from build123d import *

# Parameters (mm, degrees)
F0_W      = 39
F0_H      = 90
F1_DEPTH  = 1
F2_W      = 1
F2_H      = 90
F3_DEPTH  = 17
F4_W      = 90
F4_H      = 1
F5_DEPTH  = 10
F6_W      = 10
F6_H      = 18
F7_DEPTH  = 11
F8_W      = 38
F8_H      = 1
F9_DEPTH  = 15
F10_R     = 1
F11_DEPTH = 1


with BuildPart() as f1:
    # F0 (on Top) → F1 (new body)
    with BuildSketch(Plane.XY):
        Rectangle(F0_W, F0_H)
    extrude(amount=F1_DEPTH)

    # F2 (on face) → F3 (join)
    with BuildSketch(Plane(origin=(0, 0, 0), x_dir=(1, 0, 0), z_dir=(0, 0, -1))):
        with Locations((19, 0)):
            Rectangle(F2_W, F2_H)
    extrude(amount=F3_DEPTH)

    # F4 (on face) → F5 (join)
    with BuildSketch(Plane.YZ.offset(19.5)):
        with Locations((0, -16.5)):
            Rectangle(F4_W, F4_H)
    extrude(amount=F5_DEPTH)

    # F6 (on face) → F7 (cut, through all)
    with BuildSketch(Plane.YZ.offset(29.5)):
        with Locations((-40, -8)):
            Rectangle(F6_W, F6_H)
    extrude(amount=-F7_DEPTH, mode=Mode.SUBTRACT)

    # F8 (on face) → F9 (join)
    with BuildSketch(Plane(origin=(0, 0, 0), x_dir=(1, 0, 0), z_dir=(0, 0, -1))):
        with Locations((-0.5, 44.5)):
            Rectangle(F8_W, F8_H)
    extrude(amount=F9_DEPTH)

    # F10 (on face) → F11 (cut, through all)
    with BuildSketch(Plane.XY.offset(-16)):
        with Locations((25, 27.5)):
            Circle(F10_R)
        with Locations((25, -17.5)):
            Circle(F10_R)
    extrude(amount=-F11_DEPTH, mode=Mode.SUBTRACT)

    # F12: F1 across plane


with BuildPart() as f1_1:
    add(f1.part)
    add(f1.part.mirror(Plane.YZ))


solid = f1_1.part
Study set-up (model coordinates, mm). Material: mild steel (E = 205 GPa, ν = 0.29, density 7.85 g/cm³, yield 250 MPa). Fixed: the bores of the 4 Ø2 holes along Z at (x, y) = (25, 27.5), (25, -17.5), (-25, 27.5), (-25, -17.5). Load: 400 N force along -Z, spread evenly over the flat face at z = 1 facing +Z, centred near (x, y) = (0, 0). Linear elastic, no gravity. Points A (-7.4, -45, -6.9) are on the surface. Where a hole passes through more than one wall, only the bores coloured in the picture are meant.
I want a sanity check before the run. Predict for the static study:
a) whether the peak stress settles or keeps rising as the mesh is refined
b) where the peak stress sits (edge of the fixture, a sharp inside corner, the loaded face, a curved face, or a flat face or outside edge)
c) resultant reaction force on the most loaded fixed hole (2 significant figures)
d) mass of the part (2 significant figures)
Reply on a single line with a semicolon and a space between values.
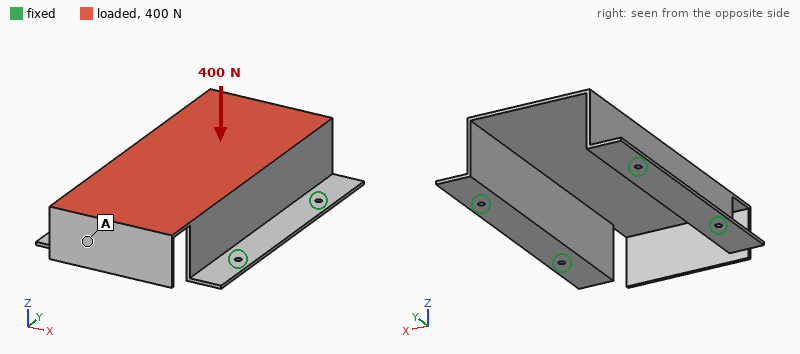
keeps rising; edge of the fixture; 130 N; 66 g
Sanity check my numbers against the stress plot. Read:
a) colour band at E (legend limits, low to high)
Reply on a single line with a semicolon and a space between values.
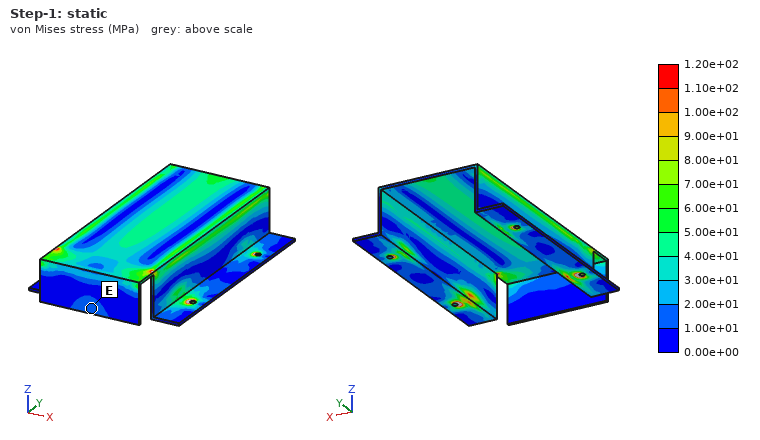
1.00e+01 to 2.00e+01 MPa
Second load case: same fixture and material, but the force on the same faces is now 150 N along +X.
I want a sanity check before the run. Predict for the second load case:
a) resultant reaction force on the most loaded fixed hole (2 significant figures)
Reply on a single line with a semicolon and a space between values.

46 N
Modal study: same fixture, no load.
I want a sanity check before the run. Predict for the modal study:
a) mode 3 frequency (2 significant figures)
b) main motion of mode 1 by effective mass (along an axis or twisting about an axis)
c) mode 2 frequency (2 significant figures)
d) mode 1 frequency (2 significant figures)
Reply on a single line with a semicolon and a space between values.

1900 Hz; along X; 1300 Hz; 1100 Hz
